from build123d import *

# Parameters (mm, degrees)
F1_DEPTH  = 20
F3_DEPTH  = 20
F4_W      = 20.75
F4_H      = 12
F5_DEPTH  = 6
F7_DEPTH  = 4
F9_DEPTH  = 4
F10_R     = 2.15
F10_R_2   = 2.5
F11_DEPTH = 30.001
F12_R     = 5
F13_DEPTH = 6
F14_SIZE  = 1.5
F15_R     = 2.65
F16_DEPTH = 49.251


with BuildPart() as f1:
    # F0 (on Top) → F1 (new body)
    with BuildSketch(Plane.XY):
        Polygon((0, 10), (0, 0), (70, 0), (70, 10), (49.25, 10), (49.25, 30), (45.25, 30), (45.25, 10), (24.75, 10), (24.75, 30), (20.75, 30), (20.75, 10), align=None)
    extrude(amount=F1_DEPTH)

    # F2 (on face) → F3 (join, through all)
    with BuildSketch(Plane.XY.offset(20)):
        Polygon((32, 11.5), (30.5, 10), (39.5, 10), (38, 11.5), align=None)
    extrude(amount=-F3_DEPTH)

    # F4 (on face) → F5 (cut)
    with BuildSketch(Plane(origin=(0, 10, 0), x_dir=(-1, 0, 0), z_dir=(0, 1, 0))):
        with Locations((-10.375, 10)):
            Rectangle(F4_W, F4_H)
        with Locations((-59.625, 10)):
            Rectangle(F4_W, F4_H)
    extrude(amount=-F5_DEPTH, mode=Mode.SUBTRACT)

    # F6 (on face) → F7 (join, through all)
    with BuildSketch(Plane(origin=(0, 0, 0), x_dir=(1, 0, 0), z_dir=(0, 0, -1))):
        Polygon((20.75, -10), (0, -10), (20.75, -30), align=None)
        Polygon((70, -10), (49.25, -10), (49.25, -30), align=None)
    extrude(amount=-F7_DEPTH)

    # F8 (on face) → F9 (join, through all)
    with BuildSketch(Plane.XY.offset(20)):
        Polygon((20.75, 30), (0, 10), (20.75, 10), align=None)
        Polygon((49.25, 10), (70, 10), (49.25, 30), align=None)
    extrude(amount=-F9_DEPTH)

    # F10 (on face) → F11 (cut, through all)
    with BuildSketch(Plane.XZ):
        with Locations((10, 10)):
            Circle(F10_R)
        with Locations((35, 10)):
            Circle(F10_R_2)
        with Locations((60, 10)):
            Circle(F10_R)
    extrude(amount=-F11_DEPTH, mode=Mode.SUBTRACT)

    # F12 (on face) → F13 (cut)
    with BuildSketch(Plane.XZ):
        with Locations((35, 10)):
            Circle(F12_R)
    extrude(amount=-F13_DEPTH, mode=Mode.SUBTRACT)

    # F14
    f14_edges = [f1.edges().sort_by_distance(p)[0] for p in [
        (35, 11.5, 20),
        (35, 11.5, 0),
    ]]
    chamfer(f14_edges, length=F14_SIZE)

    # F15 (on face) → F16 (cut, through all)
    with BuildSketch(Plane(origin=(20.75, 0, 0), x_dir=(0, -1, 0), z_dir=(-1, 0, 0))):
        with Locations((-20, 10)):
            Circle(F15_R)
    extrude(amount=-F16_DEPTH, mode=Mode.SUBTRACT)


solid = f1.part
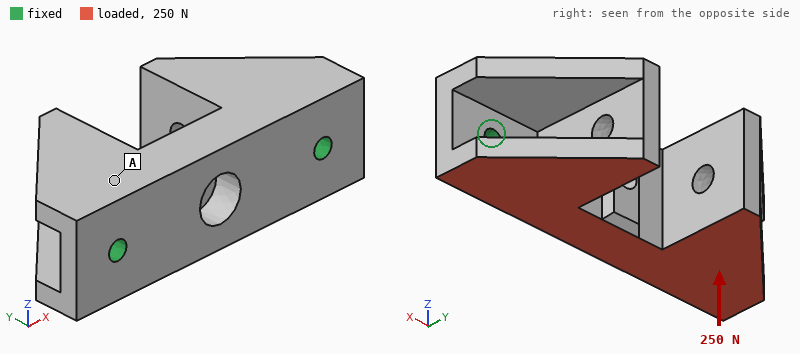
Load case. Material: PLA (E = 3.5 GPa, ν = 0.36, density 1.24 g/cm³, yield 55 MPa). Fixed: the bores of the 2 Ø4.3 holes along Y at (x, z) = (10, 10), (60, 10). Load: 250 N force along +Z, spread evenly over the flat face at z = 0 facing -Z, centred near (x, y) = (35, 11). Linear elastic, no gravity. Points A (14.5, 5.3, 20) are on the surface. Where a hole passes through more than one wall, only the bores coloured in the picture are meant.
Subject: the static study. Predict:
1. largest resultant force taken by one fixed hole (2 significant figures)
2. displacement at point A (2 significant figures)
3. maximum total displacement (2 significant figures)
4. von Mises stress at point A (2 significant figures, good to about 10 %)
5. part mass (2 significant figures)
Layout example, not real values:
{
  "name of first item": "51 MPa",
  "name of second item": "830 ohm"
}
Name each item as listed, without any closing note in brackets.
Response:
{
  "largest resultant force taken by one fixed hole": "130 N",
  "displacement at point A": "0.075 mm",
  "maximum total displacement": "0.28 mm",
  "von Mises stress at point A": "2.3 MPa",
  "part mass": "21 g"
}
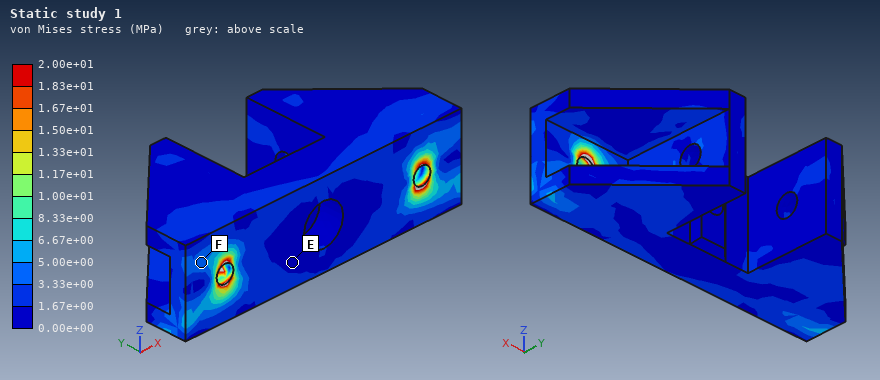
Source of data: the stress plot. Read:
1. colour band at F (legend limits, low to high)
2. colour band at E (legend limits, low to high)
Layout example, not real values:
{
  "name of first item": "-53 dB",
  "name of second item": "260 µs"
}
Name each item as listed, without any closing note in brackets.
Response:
{
  "colour band at F": "3.33e+00 to 5.00e+00 MPa",
  "colour band at E": "0.00e+00 to 1.67e+00 MPa"
}
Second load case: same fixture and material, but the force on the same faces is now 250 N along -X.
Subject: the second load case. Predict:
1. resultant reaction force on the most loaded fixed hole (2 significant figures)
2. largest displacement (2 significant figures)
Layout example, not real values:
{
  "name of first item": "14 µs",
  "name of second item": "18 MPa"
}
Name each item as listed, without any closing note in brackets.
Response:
{
  "resultant reaction force on the most loaded fixed hole": "140 N",
  "largest displacement": "49 µm"
}
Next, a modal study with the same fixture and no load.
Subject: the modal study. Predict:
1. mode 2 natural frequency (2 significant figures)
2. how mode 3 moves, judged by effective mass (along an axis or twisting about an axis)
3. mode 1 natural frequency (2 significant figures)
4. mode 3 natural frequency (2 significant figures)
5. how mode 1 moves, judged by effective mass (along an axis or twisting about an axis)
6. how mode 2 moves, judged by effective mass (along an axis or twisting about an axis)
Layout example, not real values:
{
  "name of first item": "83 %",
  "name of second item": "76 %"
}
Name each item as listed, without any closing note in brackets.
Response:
{
  "mode 2 natural frequency": "2500 Hz",
  "how mode 3 moves, judged by effective mass": "twisting about Y",
  "mode 1 natural frequency": "1400 Hz",
  "mode 3 natural frequency": "2900 Hz",
  "how mode 1 moves, judged by effective mass": "along Z",
  "how mode 2 moves, judged by effective mass": "along Y"
}
